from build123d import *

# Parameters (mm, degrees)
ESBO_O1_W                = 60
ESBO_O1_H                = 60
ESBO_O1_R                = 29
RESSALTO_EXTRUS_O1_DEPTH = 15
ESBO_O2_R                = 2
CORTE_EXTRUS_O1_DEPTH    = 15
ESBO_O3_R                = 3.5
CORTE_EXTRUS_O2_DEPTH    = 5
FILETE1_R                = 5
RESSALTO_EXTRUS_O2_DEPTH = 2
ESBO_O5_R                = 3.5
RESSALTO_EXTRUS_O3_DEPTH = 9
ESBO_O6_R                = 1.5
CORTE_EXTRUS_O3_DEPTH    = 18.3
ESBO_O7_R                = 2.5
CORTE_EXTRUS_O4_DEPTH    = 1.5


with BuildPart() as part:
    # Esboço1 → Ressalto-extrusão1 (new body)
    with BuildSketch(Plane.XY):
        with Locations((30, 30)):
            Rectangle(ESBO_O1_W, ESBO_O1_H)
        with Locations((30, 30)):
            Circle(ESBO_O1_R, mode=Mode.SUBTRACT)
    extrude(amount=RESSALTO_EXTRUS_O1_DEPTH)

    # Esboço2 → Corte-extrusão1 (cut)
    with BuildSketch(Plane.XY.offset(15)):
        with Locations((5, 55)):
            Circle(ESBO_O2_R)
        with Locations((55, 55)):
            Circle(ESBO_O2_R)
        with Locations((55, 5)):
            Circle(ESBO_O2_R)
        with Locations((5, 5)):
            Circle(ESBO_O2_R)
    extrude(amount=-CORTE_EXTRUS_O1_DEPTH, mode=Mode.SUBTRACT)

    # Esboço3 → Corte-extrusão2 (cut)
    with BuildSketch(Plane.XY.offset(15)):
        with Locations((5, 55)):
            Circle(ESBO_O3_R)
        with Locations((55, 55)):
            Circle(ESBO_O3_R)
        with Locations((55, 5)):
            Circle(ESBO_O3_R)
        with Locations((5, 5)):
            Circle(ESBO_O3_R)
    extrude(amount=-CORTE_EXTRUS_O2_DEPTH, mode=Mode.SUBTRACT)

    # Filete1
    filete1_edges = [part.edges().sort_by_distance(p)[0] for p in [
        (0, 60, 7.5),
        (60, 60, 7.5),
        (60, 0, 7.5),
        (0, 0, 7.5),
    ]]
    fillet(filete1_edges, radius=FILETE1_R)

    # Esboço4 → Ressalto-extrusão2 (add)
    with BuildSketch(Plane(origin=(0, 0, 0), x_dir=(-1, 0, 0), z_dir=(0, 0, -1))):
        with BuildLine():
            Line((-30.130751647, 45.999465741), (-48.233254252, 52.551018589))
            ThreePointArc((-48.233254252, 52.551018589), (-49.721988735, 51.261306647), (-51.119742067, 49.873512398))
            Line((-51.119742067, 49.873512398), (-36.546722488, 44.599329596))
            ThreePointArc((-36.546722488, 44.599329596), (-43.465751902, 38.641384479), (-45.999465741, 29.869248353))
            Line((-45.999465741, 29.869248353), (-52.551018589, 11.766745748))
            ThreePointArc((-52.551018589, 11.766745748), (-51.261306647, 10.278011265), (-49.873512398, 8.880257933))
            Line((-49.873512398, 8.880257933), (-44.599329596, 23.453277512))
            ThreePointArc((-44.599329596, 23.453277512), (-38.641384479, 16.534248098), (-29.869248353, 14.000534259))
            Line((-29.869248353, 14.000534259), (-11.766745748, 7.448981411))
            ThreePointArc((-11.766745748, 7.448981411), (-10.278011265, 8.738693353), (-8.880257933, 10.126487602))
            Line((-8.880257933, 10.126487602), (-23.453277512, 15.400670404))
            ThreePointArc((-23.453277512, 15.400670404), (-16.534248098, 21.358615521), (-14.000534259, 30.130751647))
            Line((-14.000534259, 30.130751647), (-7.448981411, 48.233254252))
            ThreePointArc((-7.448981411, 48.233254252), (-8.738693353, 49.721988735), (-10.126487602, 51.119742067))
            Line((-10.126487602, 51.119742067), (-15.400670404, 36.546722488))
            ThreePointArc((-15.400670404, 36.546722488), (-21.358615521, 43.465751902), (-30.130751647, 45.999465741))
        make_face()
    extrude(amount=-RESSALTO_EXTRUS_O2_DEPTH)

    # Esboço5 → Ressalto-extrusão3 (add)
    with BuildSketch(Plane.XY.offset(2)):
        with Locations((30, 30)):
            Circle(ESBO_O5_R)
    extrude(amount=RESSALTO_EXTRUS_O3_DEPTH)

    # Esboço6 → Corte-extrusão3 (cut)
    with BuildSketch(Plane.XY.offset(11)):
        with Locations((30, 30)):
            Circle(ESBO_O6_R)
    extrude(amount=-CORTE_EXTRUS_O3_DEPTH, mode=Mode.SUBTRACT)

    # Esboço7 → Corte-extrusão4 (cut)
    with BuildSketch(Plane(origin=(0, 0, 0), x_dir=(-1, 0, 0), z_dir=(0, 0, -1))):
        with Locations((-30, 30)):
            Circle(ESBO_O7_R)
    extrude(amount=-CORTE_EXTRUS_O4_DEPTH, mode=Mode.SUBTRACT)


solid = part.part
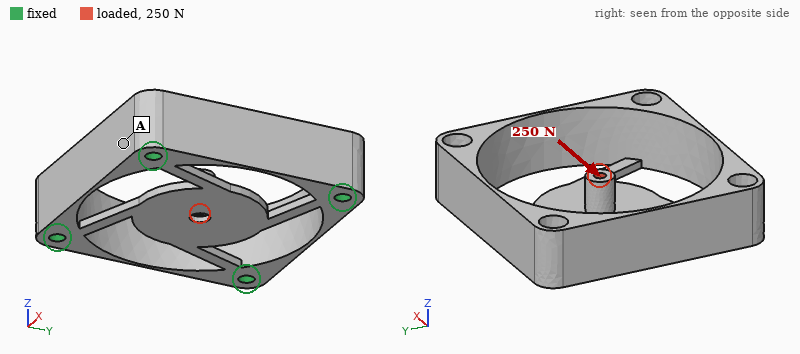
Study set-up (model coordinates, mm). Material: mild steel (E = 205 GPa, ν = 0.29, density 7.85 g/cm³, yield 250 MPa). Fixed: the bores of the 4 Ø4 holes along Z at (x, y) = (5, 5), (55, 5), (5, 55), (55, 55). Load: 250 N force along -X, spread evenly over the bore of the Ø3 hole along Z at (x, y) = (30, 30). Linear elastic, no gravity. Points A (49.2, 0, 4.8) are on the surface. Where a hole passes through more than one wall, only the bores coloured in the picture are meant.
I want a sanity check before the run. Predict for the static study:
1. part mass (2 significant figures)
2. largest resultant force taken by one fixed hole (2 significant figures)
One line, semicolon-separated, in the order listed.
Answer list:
120 g; 110 N
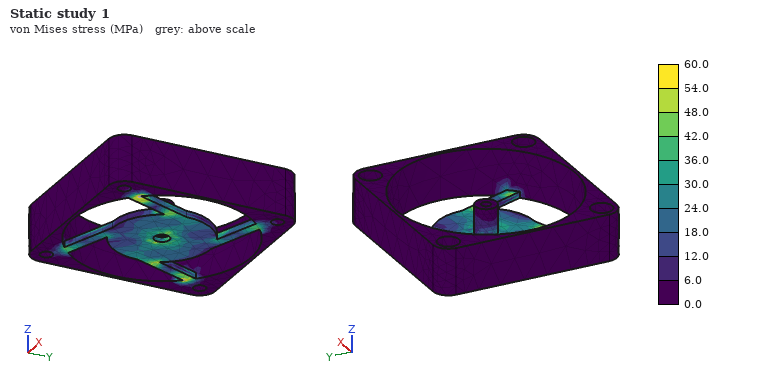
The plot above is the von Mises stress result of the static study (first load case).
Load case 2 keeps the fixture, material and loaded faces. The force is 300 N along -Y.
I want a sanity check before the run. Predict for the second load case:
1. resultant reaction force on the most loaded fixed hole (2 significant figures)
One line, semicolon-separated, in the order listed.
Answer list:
140 N
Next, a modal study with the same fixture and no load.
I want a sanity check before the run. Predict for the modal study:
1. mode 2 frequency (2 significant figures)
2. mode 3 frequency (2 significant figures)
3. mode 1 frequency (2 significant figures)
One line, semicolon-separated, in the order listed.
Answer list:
4400 Hz; 4500 Hz; 2200 Hz
